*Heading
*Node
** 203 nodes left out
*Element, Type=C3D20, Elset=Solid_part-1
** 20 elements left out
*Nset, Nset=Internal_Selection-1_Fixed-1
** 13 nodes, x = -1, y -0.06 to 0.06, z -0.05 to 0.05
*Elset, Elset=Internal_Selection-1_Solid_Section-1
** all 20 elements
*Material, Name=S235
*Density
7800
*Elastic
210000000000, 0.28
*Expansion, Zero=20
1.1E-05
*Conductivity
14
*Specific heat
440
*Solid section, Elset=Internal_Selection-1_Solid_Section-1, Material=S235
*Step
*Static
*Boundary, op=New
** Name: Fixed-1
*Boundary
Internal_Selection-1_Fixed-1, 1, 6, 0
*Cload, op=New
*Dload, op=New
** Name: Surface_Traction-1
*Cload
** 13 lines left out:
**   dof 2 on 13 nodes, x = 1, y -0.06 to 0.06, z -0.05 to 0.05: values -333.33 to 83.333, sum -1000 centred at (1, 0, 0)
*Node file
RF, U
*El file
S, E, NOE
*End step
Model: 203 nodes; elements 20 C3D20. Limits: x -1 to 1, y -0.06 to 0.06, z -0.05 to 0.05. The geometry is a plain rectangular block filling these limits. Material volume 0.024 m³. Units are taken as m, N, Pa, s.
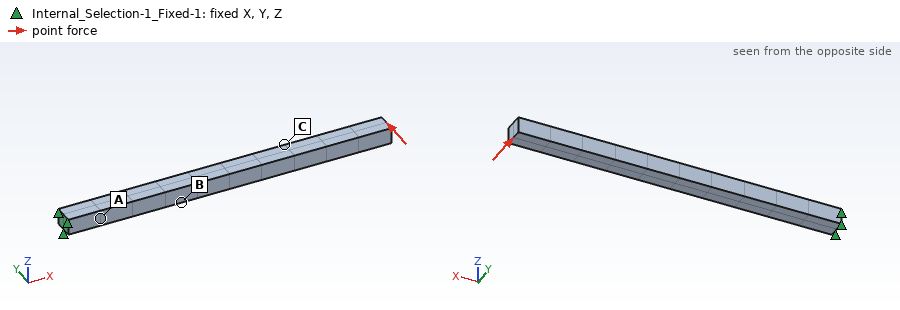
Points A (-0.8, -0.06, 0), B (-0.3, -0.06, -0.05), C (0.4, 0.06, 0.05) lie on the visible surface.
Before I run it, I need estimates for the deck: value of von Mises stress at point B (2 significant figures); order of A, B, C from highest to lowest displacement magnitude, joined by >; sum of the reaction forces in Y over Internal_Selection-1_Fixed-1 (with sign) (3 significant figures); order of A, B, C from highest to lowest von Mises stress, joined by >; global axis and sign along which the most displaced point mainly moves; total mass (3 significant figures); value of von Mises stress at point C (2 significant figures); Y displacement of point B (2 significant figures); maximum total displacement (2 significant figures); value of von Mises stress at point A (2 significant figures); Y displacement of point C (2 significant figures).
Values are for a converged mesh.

5.4e+06 Pa
C > B > A
1000 N
A > B > C
-Y
187 kg
2.5e+06 Pa
-1.4e-04 m
8.8e-04 m
7.5e+06 Pa
-5.0e-04 m
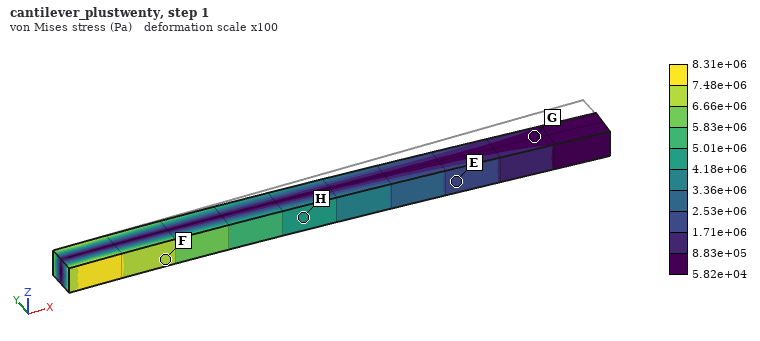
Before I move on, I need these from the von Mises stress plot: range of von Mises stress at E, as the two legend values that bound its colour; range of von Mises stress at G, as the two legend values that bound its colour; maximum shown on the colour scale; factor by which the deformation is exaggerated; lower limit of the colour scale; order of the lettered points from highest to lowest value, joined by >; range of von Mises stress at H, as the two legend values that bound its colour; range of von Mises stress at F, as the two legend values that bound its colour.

1.71e+06 to 2.53e+06 Pa
5.82e+04 to 8.83e+05 Pa
8.31e+06 Pa
100
5.82e+04 Pa
F > H > E > G
4.18e+06 to 5.01e+06 Pa
6.66e+06 to 7.48e+06 Pa
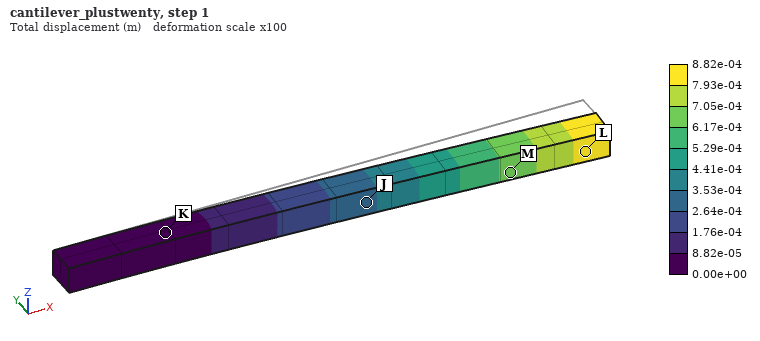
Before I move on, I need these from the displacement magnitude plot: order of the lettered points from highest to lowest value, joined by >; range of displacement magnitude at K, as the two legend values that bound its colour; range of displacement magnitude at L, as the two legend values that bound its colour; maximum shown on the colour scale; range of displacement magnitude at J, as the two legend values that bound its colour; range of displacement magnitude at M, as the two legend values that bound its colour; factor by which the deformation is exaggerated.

L > M > J > K
0.00e+00 to 8.82e-05 m
7.93e-04 to 8.82e-04 m
8.82e-04 m
2.64e-04 to 3.53e-04 m
6.17e-04 to 7.05e-04 m
100
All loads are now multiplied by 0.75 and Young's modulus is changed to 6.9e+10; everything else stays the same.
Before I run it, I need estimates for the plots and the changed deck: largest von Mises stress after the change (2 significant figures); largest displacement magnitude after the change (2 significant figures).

6.2e+06 Pa
0.0020 m
